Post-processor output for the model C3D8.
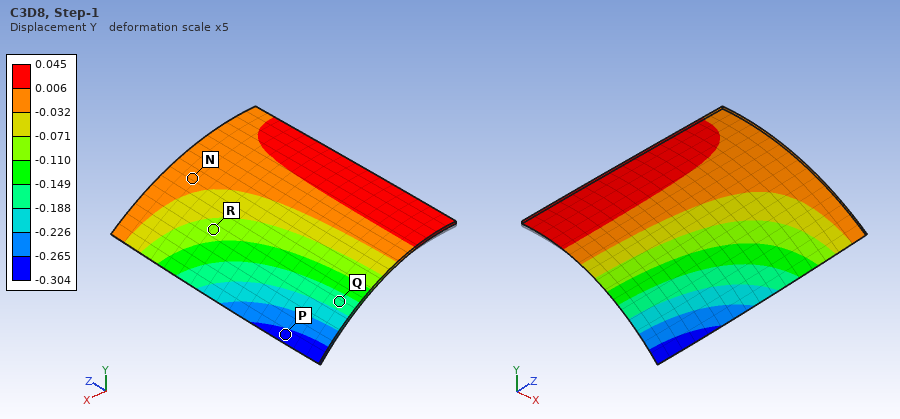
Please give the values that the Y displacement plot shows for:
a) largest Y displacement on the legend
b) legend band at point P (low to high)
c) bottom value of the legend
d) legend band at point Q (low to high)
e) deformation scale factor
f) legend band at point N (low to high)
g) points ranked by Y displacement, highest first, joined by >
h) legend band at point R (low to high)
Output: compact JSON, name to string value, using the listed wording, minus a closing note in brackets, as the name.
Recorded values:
{"largest Y displacement on the legend": "0.045", "legend band at point P": "-0.304 to -0.265", "bottom value of the legend": "-0.304", "legend band at point Q": "-0.188 to -0.149", "deformation scale factor": "5", "legend band at point N": "-0.032 to 0.006", "points ranked by Y displacement, highest first, joined by >": "N > R > Q > P", "legend band at point R": "-0.110 to -0.071"}
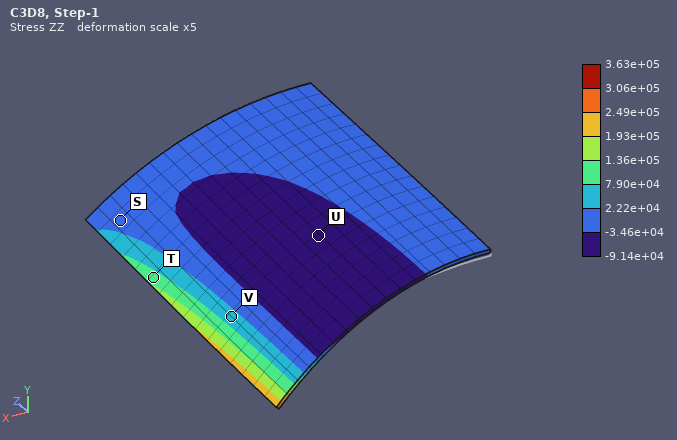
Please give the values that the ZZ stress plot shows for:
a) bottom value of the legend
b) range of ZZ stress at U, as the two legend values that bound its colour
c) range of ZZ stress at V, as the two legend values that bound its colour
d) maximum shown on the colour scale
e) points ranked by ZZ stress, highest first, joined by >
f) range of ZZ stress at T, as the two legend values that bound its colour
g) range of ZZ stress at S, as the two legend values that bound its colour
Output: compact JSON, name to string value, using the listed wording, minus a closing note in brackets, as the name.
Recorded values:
{"bottom value of the legend": "-9.14e+04", "range of ZZ stress at U, as the two legend values that bound its colour": "-9.14e+04 to -3.46e+04", "range of ZZ stress at V, as the two legend values that bound its colour": "2.22e+04 to 7.90e+04", "maximum shown on the colour scale": "3.63e+05", "points ranked by ZZ stress, highest first, joined by >": "T > V > S > U", "range of ZZ stress at T, as the two legend values that bound its colour": "7.90e+04 to 1.36e+05", "range of ZZ stress at S, as the two legend values that bound its colour": "-3.46e+04 to 2.22e+04"}
